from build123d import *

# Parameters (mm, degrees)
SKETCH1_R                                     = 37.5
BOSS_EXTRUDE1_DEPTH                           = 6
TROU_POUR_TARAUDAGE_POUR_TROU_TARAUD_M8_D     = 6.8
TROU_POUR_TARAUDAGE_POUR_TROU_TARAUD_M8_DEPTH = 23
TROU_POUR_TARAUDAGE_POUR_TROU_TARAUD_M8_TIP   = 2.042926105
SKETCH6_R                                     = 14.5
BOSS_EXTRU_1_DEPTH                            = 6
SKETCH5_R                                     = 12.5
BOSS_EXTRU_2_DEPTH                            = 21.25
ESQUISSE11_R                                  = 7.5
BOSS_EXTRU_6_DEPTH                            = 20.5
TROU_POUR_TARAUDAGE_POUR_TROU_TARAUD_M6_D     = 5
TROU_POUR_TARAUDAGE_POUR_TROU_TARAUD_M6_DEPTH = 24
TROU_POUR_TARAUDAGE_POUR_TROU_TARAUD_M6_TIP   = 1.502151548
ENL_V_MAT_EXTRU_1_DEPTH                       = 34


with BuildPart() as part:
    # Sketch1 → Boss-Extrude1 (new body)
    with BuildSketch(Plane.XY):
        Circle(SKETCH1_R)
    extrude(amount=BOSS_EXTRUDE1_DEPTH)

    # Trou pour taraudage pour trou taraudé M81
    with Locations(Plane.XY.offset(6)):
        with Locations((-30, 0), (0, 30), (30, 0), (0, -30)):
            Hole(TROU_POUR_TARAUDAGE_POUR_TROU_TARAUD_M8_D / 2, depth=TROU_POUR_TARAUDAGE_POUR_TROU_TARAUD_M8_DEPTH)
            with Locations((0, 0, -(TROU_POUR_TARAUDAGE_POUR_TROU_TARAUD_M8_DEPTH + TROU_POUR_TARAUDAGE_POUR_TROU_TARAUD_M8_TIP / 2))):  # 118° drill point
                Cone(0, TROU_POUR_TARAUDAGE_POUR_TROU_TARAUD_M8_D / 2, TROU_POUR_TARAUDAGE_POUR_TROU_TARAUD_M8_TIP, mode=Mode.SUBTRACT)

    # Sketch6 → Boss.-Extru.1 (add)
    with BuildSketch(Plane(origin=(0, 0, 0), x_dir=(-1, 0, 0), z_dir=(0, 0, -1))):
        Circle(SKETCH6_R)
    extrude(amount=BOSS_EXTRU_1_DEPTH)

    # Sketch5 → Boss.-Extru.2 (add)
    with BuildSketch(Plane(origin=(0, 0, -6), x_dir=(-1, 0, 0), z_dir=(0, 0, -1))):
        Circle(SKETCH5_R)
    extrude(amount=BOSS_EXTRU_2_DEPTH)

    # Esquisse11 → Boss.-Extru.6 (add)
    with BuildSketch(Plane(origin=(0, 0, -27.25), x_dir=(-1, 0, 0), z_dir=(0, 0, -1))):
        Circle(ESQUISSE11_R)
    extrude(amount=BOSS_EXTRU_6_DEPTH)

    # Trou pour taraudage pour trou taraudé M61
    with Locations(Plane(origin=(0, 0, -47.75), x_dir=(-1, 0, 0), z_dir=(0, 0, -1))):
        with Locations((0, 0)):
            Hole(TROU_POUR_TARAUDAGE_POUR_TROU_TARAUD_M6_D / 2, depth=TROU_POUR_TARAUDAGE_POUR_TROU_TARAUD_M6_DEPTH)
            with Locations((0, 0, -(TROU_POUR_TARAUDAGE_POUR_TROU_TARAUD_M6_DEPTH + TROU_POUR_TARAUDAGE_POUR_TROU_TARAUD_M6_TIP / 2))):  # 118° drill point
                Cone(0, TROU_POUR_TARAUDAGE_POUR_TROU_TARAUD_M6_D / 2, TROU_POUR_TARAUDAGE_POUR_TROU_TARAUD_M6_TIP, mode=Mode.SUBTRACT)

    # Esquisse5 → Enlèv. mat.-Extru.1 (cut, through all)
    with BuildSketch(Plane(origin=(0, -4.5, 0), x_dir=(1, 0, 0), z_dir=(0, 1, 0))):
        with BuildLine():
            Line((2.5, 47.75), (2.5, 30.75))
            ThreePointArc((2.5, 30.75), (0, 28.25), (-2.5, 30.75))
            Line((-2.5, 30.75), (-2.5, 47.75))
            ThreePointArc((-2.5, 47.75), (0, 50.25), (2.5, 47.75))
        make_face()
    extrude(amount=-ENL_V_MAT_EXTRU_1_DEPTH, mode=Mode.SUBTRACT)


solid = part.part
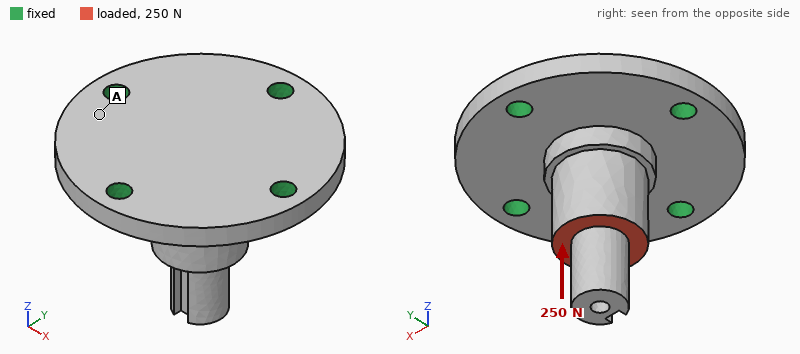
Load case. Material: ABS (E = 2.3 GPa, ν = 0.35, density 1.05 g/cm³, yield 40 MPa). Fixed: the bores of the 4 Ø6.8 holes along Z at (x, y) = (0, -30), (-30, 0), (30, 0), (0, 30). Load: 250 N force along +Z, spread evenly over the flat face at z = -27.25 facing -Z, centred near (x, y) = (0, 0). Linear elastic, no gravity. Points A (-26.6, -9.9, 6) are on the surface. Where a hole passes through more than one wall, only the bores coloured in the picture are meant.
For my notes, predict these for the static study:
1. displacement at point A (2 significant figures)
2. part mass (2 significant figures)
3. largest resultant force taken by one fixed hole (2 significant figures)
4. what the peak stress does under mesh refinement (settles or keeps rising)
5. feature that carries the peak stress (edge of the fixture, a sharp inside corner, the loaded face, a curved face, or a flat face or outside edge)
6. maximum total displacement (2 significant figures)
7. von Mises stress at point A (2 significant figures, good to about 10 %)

7.1 µm
45 g
65 N
keeps rising
edge of the fixture
42 µm
0.84 MPa
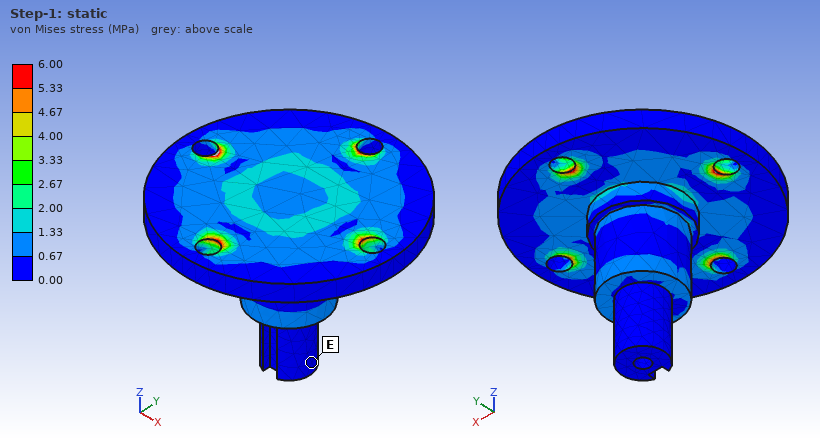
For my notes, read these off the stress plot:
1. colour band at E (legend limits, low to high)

0.00 to 0.67 MPa
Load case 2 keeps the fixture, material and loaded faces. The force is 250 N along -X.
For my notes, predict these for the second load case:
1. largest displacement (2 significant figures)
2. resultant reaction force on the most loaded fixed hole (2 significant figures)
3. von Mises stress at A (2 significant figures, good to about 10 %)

0.28 mm
170 N
1.3 MPa
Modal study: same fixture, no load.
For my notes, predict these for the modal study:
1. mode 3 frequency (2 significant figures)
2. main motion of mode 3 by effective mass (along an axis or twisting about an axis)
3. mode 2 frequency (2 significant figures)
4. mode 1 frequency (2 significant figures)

2600 Hz
along Z
1800 Hz
1800 Hz
